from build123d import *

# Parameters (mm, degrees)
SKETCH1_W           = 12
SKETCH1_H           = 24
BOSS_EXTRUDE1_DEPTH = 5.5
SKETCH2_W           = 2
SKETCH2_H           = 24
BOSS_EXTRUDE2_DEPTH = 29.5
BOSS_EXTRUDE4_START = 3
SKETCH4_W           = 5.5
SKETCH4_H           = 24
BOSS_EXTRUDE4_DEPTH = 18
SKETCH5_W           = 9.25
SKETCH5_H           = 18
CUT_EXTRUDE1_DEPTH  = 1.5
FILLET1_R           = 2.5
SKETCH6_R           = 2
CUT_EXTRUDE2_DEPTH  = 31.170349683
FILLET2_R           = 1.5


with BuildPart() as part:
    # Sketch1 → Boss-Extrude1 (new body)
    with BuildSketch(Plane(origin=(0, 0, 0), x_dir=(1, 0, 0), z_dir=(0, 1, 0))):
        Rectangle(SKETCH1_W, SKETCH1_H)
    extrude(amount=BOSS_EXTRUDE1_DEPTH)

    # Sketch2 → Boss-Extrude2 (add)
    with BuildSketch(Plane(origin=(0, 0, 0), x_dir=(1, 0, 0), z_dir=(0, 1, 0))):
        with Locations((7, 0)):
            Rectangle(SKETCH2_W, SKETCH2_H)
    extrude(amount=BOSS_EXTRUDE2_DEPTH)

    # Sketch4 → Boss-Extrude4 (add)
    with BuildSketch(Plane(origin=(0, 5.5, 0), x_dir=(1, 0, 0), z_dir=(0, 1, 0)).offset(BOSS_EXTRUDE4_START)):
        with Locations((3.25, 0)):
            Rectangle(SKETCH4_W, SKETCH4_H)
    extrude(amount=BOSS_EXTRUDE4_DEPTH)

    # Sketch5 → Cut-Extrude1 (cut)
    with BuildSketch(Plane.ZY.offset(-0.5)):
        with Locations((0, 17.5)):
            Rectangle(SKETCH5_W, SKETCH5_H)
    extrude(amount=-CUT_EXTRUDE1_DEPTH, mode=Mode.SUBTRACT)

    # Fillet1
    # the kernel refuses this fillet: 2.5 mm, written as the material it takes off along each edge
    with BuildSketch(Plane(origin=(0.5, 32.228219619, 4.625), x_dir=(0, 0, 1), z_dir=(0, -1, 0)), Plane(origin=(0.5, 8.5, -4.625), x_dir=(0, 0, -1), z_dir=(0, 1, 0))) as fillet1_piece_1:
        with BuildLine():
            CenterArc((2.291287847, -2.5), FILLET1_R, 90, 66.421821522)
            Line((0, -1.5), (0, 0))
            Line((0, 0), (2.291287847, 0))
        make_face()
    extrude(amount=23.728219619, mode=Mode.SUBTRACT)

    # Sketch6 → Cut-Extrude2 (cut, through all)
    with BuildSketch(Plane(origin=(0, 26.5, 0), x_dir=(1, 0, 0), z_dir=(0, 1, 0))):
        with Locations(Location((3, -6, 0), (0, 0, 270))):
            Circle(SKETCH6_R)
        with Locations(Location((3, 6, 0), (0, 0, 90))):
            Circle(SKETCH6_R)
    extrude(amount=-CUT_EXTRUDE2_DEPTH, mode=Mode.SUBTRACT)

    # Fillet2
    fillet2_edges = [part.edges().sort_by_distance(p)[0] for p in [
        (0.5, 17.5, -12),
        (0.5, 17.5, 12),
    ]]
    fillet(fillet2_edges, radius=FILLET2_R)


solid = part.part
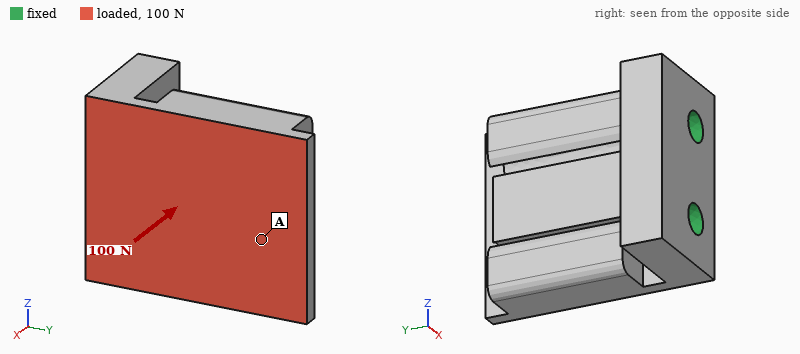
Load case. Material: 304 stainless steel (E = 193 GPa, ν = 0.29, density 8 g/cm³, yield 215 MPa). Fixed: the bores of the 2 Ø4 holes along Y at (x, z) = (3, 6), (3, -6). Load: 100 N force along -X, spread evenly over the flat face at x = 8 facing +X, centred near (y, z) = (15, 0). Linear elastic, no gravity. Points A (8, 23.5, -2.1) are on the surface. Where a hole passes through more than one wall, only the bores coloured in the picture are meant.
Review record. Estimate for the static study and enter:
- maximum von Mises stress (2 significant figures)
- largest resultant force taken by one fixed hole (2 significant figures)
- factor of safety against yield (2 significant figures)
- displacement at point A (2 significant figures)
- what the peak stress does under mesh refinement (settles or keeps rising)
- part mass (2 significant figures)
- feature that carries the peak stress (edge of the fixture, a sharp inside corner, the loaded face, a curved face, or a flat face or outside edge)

54 MPa
50 N
4.0
24 µm
settles
36 g
the loaded face
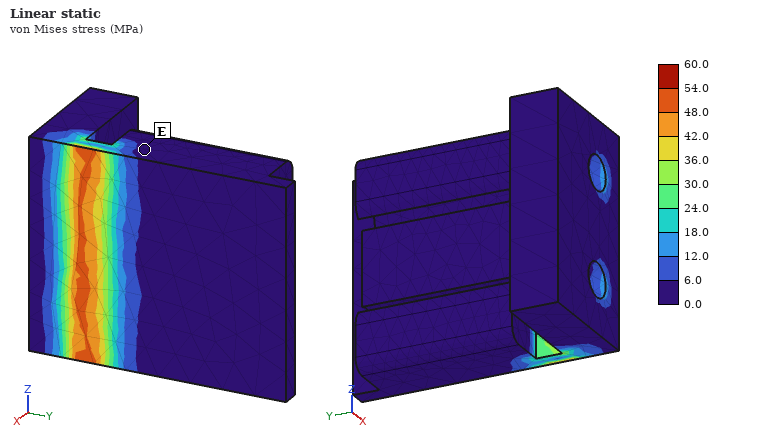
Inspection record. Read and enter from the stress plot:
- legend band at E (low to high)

0.0 to 6.0 MPa
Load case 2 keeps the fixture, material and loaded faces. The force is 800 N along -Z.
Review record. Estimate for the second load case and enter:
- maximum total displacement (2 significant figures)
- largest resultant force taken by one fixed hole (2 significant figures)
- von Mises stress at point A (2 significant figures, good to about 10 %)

11 µm
720 N
13 MPa
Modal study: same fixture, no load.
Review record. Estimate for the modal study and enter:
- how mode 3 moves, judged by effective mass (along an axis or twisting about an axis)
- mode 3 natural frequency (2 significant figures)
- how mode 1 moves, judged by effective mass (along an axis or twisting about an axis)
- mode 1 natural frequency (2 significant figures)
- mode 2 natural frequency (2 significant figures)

along Z
11 kHz
along X
2100 Hz
8600 Hz
